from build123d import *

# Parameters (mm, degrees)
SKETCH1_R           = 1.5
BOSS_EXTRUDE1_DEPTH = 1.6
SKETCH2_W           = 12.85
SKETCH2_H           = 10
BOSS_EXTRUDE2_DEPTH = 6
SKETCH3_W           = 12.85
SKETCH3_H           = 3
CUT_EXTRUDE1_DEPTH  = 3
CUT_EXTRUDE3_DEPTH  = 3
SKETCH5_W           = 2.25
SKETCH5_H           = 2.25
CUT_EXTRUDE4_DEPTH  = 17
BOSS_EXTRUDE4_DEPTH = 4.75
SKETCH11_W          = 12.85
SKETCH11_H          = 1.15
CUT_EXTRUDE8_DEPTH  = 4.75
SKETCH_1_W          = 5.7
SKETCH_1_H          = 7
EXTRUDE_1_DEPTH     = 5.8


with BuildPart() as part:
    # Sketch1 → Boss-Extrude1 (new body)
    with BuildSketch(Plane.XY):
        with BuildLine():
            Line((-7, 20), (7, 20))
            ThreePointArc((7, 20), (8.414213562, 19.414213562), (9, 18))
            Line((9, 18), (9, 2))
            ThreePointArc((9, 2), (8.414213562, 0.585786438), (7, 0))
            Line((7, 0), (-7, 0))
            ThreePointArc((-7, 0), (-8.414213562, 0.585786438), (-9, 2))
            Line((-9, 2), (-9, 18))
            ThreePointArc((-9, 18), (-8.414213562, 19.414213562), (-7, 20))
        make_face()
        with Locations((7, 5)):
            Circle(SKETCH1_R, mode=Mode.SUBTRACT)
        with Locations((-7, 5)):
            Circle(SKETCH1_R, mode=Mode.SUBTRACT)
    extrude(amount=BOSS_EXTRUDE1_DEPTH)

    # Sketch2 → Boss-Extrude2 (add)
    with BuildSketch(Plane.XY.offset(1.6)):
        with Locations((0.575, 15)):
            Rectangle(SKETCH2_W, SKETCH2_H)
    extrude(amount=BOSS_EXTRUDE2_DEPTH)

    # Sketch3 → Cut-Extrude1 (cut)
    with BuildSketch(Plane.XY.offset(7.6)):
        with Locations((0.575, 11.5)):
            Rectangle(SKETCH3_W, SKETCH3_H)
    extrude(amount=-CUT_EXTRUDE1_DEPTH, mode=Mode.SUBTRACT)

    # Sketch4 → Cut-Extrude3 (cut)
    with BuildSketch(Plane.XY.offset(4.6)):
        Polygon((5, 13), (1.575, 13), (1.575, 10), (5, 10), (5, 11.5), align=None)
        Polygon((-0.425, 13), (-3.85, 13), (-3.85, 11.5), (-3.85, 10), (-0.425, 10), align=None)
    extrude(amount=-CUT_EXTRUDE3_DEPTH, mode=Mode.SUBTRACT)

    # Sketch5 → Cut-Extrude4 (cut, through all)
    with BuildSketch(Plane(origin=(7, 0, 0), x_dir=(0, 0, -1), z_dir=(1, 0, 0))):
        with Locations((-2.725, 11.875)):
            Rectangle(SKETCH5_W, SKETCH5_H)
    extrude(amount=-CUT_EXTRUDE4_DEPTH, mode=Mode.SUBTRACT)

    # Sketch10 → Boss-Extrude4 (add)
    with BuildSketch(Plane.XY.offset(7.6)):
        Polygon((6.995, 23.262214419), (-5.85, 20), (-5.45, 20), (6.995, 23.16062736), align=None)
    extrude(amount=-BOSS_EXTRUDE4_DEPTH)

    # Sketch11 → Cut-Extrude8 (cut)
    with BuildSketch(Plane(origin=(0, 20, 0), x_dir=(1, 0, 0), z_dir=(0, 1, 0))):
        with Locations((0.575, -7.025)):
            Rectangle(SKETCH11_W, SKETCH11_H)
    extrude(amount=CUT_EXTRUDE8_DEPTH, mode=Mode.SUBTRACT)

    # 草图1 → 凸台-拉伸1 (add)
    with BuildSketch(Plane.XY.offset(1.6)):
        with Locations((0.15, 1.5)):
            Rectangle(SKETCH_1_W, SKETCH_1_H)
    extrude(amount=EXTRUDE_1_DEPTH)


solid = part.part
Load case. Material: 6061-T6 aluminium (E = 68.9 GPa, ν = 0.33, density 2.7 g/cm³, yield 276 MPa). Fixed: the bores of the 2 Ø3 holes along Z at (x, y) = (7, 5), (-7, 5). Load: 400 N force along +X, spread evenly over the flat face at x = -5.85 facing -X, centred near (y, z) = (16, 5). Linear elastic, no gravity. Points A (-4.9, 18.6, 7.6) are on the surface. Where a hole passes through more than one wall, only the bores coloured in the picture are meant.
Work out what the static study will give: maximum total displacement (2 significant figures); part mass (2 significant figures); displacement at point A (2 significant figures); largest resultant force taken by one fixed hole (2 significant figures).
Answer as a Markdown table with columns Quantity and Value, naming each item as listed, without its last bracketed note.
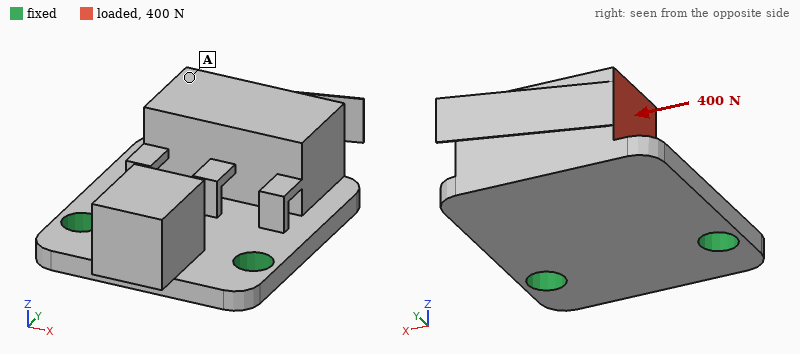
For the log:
| Quantity | Value |
|---|---|
| maximum total displacement | 46 µm |
| part mass | 3.6 g |
| displacement at point A | 41 µm |
| largest resultant force taken by one fixed hole | 370 N |
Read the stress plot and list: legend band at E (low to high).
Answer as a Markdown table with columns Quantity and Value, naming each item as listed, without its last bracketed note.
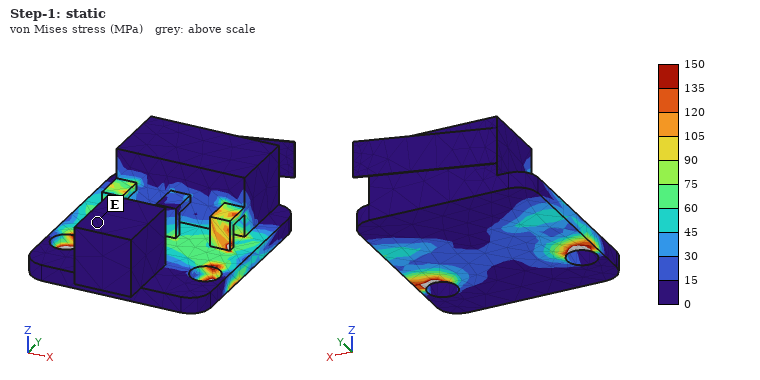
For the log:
| Quantity | Value |
|---|---|
| legend band at E | 0 to 15 MPa |
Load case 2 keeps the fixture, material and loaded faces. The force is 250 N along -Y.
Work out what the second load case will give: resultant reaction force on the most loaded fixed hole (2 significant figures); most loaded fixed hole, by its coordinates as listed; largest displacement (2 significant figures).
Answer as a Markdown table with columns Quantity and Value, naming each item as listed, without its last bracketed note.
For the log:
| Quantity | Value |
|---|---|
| resultant reaction force on the most loaded fixed hole | 230 N |
| most loaded fixed hole, by its coordinates as listed | (-7, 5) |
| largest displacement | 0.22 mm |
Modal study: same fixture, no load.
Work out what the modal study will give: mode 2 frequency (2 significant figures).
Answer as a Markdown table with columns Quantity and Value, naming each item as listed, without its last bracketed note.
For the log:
| Quantity | Value |
|---|---|
| mode 2 frequency | 3200 Hz |
